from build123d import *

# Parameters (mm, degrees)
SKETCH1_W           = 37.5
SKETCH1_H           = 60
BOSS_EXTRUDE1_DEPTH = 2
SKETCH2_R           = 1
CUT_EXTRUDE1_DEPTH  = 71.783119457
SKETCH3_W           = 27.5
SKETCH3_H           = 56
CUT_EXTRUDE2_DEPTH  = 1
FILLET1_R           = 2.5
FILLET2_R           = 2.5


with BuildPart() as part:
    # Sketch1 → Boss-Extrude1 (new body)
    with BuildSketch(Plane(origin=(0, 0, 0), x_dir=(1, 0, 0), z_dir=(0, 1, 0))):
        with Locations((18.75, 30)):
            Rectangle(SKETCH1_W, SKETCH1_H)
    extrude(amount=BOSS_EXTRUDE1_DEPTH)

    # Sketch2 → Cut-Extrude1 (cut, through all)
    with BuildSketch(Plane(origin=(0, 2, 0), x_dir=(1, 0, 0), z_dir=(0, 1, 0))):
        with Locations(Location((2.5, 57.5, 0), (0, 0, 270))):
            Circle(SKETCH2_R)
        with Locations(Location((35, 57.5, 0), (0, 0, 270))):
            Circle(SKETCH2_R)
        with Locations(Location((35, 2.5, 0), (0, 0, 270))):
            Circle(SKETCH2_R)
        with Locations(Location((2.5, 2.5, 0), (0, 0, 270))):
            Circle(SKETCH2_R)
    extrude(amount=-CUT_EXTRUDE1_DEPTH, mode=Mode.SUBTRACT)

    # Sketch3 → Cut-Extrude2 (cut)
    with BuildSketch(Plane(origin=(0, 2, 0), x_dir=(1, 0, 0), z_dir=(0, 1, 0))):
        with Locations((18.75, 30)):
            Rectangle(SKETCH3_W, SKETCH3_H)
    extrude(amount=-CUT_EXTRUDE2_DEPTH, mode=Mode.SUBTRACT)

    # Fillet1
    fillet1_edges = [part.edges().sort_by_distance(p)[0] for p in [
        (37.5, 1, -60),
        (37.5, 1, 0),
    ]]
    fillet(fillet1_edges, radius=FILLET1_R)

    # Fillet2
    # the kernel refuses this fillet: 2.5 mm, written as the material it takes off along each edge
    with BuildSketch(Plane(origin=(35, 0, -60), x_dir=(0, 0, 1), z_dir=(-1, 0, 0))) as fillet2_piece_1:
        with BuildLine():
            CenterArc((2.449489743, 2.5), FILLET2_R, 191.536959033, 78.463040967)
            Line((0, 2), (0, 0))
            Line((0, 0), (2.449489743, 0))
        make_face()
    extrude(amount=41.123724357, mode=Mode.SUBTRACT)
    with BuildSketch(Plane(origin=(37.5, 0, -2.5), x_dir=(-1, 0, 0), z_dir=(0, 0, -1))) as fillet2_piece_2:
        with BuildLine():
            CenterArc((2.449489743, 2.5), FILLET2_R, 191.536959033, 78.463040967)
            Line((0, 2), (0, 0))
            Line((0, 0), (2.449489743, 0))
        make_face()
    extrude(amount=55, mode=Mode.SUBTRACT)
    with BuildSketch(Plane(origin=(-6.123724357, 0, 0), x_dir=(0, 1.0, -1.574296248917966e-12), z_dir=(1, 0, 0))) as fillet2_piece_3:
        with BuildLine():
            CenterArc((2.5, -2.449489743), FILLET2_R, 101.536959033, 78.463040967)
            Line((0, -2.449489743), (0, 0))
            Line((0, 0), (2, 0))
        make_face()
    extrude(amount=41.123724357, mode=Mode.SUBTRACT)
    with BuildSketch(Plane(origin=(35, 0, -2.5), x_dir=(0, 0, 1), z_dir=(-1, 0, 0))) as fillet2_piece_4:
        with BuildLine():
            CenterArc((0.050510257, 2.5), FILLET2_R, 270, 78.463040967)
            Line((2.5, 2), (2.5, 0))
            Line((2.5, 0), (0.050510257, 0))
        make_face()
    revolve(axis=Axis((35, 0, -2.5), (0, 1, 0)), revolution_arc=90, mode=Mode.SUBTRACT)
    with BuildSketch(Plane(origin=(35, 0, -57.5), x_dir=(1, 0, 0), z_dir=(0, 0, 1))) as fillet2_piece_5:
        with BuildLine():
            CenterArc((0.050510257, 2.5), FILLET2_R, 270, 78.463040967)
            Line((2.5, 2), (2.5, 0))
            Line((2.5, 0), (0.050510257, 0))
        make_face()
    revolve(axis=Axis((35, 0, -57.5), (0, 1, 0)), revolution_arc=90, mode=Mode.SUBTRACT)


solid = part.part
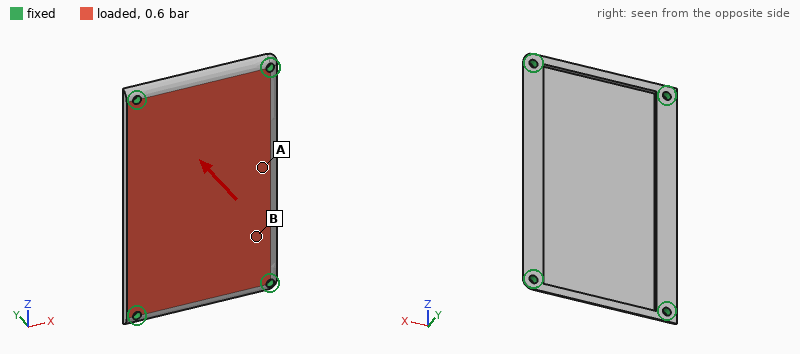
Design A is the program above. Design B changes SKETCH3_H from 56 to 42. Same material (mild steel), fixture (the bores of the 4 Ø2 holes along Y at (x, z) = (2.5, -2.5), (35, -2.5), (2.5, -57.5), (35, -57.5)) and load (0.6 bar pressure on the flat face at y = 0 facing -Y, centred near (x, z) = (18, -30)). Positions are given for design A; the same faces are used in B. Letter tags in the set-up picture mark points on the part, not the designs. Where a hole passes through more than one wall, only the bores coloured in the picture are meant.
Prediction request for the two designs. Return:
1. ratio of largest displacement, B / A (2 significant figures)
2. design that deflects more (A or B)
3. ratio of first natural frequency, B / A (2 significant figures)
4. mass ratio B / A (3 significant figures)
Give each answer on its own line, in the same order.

0.81
A
1.1
1.14
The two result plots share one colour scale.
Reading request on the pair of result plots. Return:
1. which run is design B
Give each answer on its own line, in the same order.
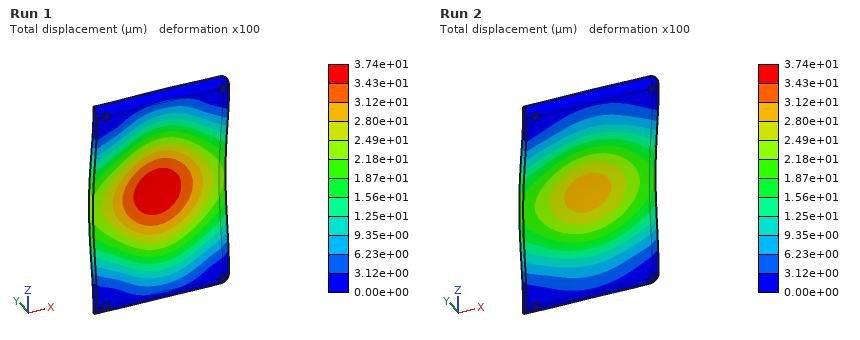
Run 2
